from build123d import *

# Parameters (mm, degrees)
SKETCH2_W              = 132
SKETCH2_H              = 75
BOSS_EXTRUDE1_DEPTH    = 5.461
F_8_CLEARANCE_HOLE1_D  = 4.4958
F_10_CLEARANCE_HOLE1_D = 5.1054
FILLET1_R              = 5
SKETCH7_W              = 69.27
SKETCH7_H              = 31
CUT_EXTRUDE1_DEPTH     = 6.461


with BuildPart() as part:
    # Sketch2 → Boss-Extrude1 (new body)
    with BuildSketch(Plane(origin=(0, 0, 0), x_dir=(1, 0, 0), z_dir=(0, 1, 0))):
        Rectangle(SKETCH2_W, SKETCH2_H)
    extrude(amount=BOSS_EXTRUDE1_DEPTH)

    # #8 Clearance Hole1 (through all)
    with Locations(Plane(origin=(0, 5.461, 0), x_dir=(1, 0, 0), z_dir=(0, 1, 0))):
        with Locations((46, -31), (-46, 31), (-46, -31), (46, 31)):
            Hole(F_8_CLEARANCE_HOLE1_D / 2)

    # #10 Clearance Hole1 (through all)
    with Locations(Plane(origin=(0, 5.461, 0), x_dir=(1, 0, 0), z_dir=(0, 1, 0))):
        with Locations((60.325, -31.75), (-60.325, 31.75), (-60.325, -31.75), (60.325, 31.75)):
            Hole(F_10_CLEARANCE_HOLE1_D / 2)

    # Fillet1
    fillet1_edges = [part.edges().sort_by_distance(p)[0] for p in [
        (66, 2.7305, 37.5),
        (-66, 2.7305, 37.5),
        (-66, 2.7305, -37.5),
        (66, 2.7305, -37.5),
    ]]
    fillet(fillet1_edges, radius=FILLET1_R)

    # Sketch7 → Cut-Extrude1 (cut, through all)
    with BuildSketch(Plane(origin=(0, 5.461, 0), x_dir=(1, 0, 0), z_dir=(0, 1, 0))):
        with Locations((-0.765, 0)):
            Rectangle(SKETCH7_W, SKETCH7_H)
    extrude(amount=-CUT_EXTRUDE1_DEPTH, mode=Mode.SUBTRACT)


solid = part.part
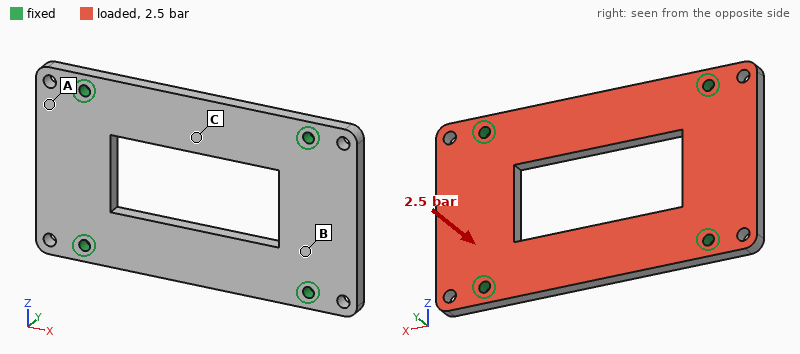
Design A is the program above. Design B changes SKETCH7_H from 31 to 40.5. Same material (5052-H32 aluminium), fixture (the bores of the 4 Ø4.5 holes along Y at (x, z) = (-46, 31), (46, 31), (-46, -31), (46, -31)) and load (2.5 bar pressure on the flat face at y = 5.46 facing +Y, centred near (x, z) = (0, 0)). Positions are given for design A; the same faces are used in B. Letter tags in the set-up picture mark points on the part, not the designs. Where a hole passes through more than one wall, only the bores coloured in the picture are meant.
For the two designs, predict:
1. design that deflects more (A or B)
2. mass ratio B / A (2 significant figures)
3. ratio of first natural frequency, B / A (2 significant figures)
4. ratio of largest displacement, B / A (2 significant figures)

A
0.91
1.1
0.83
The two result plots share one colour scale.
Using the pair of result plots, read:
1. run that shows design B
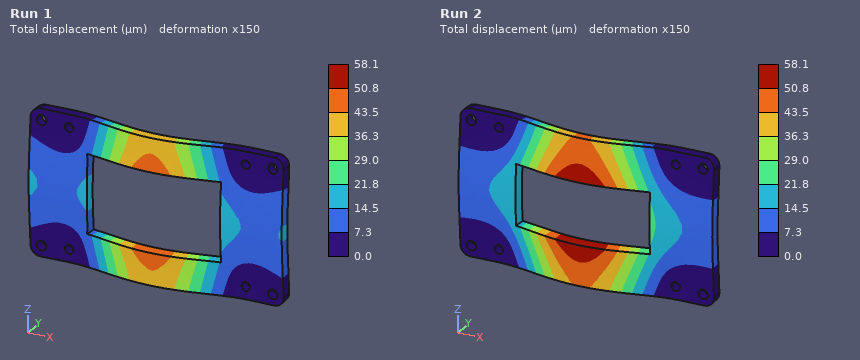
Run 1
